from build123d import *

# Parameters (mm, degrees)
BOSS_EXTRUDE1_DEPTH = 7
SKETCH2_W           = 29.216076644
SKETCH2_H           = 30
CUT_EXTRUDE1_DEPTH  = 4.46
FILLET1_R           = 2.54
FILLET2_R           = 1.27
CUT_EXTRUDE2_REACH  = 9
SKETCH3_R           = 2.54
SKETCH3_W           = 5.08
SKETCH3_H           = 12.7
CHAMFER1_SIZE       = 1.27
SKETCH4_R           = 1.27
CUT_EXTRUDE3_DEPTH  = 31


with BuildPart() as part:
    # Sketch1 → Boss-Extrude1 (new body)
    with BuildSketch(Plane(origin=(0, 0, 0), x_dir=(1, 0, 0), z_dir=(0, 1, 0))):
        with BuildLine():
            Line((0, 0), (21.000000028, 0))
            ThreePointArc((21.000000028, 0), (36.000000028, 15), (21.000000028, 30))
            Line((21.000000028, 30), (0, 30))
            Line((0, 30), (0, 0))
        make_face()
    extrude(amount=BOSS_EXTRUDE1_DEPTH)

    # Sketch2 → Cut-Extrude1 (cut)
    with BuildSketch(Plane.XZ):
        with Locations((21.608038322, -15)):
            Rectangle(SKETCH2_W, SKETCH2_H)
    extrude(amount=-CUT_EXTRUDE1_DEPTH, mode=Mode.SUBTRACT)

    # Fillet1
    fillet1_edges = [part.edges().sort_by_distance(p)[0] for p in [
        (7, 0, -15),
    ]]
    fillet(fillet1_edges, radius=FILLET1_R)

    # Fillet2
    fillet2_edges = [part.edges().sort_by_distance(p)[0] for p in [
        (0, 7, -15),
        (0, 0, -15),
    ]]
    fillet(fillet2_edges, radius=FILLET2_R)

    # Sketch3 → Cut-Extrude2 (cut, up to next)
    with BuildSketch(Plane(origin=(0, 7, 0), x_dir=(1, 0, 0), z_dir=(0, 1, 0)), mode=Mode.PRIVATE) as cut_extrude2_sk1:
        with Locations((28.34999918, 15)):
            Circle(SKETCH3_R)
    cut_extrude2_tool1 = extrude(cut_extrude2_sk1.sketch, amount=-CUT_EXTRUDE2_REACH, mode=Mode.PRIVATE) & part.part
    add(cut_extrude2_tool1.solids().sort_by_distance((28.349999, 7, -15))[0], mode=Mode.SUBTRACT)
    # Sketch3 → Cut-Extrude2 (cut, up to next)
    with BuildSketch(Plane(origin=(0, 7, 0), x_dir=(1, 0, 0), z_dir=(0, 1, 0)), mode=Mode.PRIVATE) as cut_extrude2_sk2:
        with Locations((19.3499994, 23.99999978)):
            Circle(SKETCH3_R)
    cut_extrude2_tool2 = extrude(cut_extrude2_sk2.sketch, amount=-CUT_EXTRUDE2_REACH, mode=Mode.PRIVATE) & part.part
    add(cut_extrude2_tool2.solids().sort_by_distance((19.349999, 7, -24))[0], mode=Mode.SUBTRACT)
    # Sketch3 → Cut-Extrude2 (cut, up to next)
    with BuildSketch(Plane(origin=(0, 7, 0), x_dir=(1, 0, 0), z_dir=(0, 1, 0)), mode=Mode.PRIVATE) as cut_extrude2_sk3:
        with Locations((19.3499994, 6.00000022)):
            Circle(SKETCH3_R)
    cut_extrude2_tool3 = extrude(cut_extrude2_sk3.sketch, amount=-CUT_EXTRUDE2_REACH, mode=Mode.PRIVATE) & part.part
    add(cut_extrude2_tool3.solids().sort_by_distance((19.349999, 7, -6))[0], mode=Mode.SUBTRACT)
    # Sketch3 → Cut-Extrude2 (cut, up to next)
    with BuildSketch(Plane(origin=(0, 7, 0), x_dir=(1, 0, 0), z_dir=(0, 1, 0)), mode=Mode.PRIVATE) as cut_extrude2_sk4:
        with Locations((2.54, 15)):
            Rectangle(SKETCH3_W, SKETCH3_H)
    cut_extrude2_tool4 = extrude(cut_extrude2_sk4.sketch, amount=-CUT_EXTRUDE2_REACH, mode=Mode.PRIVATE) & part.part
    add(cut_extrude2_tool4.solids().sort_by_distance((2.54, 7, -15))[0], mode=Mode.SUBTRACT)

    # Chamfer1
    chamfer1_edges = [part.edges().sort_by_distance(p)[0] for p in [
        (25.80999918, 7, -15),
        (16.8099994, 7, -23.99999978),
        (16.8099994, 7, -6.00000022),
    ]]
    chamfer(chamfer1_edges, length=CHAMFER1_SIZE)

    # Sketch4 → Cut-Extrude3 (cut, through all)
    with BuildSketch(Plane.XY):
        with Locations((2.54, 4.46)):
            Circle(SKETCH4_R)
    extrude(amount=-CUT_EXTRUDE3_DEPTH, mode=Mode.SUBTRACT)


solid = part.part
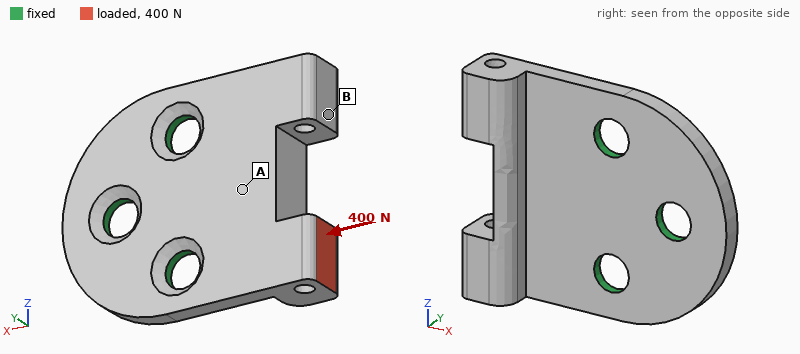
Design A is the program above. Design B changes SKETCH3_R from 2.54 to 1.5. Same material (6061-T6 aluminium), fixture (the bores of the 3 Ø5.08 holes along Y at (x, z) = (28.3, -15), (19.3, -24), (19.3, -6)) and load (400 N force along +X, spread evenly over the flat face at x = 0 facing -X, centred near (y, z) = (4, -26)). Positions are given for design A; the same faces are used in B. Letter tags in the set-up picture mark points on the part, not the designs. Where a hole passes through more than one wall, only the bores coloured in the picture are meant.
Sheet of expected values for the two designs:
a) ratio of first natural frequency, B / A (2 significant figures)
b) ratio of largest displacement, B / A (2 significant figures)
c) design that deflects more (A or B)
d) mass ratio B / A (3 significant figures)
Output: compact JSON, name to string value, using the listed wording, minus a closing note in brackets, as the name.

{"ratio of first natural frequency, B / A": "0.89", "ratio of largest displacement, B / A": "1.1", "design that deflects more": "B", "mass ratio B / A": "1.04"}
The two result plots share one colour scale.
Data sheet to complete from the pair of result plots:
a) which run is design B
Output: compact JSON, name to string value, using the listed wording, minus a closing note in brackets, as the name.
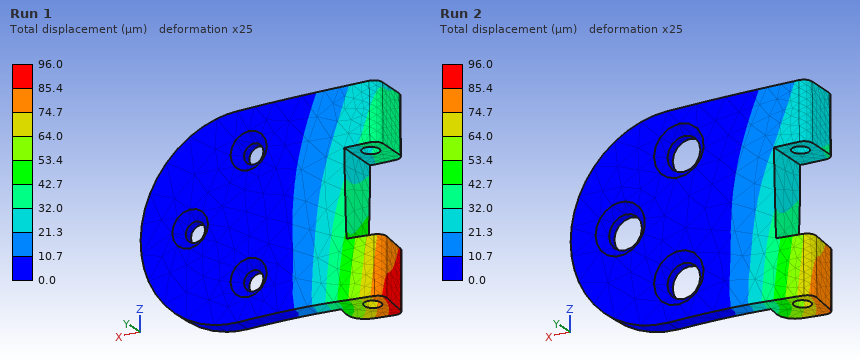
{"which run is design B": "Run 1"}
